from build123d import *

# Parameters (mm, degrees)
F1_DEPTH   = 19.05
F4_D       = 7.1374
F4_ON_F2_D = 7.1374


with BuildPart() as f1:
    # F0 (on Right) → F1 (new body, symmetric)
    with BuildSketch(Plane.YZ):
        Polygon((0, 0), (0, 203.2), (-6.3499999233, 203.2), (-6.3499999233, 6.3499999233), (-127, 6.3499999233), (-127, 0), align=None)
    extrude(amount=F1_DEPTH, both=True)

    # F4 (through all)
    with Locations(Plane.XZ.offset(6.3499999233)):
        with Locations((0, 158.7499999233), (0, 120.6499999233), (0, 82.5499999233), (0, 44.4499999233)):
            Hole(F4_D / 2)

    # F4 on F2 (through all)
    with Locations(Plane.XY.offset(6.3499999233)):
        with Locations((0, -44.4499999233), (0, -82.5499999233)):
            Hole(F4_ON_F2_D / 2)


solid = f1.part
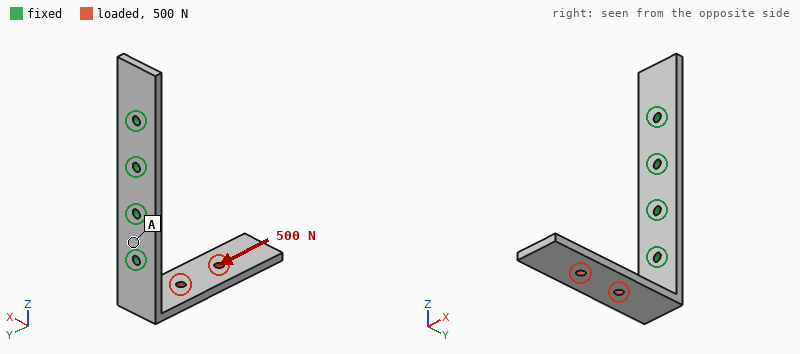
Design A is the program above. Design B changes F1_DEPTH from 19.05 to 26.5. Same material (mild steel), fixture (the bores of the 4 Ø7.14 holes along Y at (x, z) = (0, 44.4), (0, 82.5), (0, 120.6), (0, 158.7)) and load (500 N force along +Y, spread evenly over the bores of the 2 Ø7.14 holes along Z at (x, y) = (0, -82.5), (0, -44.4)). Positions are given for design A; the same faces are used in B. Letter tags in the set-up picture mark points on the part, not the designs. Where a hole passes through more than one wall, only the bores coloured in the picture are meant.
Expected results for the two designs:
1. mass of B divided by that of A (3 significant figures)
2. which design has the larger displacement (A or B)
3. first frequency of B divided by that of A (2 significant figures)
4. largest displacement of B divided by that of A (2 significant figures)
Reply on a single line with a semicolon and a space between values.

1.40; A; 0.99; 0.76
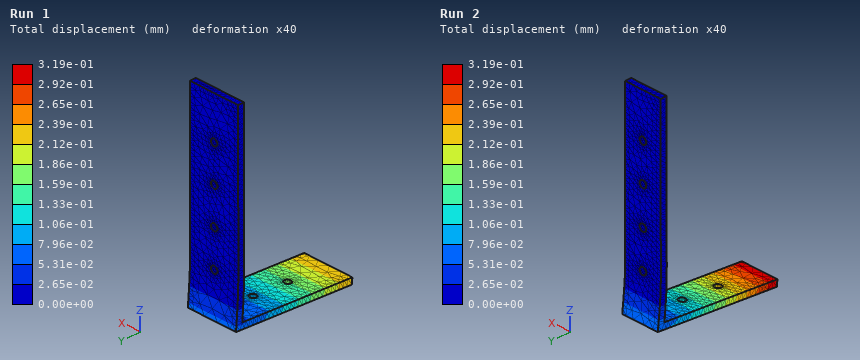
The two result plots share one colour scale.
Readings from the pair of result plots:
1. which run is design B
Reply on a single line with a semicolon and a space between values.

Run 1
